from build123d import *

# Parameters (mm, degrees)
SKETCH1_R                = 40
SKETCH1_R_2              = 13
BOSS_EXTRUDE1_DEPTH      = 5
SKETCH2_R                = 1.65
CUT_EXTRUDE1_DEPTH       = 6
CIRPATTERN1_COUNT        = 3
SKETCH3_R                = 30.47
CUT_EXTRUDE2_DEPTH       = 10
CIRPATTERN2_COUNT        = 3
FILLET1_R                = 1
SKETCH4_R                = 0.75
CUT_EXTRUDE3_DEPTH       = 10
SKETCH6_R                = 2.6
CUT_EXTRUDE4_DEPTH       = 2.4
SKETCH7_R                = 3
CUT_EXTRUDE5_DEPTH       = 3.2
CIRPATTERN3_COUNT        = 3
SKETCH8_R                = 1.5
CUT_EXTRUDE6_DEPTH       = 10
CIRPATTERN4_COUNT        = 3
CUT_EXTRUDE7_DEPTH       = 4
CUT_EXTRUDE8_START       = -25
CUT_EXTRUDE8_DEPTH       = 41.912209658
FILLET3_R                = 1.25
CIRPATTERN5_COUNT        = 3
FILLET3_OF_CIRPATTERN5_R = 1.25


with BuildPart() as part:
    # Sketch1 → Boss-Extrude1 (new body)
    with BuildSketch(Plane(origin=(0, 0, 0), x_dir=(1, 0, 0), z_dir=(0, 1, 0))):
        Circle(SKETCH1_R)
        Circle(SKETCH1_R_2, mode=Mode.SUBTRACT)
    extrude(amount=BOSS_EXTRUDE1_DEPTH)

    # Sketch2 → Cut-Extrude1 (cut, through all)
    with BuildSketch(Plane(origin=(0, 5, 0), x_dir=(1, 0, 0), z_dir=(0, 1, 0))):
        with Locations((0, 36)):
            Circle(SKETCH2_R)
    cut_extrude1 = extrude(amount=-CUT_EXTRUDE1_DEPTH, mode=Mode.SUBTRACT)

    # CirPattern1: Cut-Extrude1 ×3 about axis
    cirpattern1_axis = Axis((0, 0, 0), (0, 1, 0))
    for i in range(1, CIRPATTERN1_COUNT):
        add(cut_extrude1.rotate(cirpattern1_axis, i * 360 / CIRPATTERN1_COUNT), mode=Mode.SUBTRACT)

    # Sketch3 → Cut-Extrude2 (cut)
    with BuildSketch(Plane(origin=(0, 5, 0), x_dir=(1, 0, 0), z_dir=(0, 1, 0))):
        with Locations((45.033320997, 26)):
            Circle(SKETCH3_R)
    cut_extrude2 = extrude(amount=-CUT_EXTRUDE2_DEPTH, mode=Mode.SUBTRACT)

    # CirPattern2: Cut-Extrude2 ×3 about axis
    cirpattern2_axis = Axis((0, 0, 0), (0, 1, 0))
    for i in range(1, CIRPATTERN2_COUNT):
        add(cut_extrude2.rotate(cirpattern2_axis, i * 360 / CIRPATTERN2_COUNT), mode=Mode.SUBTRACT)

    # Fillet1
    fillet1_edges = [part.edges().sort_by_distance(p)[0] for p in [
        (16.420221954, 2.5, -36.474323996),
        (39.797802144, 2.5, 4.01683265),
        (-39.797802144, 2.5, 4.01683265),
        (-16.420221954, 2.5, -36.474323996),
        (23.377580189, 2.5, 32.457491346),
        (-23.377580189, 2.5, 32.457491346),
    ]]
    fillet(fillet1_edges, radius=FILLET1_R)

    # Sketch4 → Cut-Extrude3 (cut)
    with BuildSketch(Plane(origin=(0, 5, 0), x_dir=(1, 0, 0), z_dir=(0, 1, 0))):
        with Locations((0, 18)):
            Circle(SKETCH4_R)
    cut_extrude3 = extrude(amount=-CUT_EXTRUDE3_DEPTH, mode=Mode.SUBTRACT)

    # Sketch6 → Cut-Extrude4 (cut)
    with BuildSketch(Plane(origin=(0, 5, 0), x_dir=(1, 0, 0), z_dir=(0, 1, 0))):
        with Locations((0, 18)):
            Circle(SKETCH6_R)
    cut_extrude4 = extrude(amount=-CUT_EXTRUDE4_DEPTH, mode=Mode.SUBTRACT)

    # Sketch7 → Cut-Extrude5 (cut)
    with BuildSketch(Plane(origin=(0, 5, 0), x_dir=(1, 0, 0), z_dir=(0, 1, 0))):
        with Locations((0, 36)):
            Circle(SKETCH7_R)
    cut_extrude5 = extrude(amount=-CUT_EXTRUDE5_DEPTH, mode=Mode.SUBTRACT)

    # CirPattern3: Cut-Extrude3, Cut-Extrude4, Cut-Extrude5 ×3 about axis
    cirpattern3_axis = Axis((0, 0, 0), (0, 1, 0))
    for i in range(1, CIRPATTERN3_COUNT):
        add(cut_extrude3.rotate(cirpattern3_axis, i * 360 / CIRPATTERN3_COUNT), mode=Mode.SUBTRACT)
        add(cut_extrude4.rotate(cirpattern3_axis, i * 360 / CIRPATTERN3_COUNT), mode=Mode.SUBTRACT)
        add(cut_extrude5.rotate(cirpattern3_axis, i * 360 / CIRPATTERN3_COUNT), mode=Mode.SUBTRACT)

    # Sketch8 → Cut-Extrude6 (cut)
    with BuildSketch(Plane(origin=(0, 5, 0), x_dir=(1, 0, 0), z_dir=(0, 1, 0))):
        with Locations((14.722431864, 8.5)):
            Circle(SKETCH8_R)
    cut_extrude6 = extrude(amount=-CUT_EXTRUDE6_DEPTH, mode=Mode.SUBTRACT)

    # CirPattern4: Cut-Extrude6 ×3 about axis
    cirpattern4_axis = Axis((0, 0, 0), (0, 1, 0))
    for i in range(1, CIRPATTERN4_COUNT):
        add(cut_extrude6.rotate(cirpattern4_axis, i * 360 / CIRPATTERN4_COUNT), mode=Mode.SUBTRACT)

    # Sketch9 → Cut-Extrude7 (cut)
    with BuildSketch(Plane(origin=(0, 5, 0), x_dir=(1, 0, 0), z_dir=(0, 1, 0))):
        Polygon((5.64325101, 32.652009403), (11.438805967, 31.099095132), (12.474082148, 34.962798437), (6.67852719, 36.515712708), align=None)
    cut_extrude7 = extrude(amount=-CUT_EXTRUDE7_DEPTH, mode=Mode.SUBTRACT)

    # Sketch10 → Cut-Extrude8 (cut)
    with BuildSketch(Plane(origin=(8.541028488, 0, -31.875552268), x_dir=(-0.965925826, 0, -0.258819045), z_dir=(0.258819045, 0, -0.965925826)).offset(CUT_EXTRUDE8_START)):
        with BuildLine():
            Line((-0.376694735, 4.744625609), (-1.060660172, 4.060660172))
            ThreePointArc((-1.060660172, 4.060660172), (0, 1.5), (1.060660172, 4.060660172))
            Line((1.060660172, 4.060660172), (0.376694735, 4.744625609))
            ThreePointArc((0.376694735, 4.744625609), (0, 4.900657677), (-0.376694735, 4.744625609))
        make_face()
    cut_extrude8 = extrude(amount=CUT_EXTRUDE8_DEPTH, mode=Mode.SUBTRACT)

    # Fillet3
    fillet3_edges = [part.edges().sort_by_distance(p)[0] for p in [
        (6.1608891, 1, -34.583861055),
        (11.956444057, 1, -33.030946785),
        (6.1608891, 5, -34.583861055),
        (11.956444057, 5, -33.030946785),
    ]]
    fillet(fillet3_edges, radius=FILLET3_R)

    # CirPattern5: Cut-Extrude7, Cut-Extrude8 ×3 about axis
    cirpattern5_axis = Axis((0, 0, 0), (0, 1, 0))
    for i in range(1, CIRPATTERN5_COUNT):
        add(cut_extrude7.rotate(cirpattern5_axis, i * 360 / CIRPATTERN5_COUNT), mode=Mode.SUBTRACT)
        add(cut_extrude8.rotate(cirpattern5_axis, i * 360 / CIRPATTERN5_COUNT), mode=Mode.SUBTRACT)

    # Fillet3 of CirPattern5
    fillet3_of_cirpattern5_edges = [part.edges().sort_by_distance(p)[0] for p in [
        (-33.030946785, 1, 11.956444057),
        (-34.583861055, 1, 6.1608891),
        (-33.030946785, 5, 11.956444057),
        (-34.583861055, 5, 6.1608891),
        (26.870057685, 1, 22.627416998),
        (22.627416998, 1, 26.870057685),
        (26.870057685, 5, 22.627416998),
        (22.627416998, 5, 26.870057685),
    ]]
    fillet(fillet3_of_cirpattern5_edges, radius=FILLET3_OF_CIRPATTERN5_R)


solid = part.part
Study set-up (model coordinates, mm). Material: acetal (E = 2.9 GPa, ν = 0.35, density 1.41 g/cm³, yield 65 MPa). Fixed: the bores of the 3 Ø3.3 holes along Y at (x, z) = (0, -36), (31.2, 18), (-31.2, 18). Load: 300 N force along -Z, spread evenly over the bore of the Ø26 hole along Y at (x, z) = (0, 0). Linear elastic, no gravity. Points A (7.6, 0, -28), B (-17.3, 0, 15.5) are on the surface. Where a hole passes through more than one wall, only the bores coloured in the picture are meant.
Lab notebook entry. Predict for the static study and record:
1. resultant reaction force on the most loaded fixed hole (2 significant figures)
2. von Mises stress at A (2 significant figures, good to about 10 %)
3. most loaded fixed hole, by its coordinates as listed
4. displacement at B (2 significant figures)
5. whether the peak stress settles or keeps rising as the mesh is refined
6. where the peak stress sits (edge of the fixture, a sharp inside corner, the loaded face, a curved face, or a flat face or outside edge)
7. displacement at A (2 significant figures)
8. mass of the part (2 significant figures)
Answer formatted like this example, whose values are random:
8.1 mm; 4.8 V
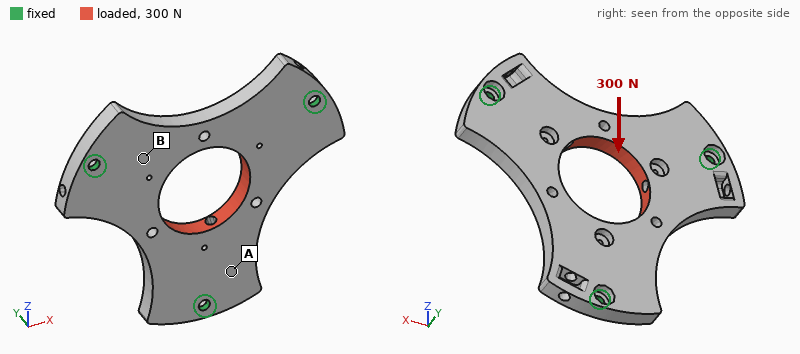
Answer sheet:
140 N; 3.3 MPa; (0, -36); 45 µm; keeps rising; a sharp inside corner; 18 µm; 17 g
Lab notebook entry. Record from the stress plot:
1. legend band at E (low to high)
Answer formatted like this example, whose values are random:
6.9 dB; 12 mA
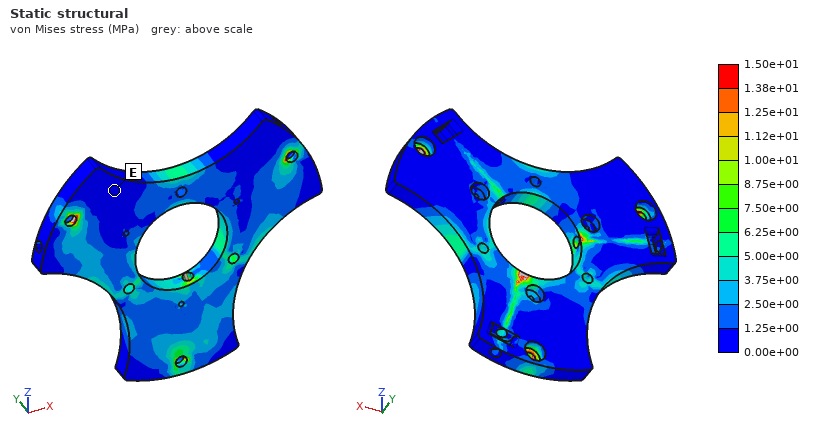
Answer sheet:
0.00e+00 to 1.25e+00 MPa
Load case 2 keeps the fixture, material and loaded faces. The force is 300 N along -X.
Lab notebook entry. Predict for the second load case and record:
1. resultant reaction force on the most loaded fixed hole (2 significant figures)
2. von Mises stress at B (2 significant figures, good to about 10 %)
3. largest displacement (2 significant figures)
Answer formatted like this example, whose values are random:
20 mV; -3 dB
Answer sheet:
130 N; 2.1 MPa; 86 µm
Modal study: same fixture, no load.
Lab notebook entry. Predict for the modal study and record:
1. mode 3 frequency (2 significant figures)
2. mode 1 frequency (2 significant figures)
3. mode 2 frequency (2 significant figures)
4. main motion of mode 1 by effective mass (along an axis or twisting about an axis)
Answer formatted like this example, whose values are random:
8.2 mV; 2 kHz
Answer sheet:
1600 Hz; 1200 Hz; 1600 Hz; along Y
